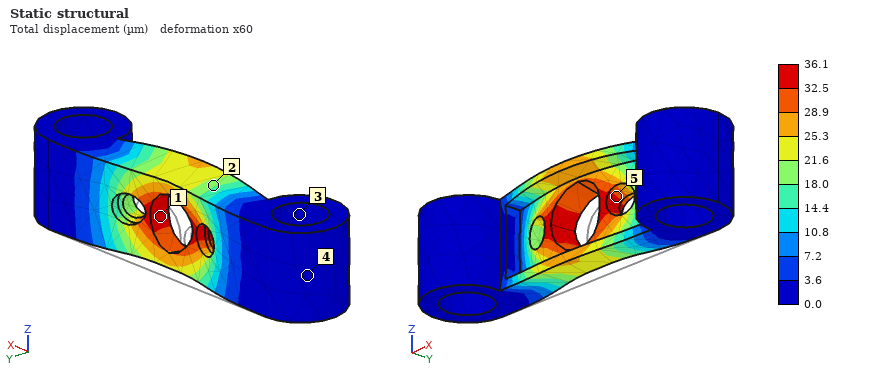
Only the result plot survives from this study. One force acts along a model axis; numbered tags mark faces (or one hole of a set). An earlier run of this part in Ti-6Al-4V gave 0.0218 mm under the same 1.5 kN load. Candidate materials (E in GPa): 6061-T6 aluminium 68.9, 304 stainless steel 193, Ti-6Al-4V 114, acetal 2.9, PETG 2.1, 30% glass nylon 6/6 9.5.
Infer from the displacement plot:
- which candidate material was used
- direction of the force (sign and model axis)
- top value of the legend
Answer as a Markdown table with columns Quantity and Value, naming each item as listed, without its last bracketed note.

| Quantity | Value |
|---|---|
| which candidate material was used | 6061-T6 aluminium |
| direction of the force | -Y |
| top value of the legend | 36.1 µm |
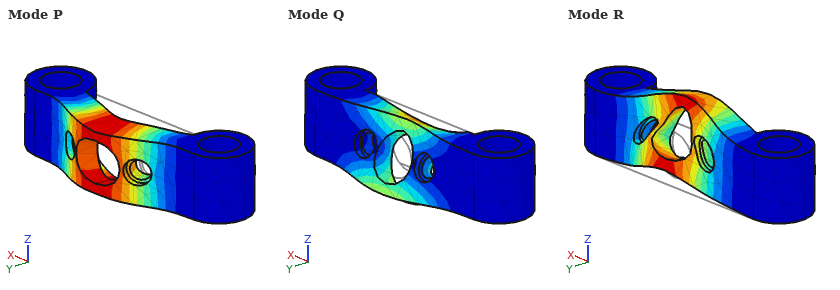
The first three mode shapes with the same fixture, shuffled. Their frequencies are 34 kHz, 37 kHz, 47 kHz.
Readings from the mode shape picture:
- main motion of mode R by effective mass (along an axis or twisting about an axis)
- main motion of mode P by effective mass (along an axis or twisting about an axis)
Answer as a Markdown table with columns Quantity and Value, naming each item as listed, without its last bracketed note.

| Quantity | Value |
|---|---|
| main motion of mode R by effective mass | along Z |
| main motion of mode P by effective mass | along Y |
